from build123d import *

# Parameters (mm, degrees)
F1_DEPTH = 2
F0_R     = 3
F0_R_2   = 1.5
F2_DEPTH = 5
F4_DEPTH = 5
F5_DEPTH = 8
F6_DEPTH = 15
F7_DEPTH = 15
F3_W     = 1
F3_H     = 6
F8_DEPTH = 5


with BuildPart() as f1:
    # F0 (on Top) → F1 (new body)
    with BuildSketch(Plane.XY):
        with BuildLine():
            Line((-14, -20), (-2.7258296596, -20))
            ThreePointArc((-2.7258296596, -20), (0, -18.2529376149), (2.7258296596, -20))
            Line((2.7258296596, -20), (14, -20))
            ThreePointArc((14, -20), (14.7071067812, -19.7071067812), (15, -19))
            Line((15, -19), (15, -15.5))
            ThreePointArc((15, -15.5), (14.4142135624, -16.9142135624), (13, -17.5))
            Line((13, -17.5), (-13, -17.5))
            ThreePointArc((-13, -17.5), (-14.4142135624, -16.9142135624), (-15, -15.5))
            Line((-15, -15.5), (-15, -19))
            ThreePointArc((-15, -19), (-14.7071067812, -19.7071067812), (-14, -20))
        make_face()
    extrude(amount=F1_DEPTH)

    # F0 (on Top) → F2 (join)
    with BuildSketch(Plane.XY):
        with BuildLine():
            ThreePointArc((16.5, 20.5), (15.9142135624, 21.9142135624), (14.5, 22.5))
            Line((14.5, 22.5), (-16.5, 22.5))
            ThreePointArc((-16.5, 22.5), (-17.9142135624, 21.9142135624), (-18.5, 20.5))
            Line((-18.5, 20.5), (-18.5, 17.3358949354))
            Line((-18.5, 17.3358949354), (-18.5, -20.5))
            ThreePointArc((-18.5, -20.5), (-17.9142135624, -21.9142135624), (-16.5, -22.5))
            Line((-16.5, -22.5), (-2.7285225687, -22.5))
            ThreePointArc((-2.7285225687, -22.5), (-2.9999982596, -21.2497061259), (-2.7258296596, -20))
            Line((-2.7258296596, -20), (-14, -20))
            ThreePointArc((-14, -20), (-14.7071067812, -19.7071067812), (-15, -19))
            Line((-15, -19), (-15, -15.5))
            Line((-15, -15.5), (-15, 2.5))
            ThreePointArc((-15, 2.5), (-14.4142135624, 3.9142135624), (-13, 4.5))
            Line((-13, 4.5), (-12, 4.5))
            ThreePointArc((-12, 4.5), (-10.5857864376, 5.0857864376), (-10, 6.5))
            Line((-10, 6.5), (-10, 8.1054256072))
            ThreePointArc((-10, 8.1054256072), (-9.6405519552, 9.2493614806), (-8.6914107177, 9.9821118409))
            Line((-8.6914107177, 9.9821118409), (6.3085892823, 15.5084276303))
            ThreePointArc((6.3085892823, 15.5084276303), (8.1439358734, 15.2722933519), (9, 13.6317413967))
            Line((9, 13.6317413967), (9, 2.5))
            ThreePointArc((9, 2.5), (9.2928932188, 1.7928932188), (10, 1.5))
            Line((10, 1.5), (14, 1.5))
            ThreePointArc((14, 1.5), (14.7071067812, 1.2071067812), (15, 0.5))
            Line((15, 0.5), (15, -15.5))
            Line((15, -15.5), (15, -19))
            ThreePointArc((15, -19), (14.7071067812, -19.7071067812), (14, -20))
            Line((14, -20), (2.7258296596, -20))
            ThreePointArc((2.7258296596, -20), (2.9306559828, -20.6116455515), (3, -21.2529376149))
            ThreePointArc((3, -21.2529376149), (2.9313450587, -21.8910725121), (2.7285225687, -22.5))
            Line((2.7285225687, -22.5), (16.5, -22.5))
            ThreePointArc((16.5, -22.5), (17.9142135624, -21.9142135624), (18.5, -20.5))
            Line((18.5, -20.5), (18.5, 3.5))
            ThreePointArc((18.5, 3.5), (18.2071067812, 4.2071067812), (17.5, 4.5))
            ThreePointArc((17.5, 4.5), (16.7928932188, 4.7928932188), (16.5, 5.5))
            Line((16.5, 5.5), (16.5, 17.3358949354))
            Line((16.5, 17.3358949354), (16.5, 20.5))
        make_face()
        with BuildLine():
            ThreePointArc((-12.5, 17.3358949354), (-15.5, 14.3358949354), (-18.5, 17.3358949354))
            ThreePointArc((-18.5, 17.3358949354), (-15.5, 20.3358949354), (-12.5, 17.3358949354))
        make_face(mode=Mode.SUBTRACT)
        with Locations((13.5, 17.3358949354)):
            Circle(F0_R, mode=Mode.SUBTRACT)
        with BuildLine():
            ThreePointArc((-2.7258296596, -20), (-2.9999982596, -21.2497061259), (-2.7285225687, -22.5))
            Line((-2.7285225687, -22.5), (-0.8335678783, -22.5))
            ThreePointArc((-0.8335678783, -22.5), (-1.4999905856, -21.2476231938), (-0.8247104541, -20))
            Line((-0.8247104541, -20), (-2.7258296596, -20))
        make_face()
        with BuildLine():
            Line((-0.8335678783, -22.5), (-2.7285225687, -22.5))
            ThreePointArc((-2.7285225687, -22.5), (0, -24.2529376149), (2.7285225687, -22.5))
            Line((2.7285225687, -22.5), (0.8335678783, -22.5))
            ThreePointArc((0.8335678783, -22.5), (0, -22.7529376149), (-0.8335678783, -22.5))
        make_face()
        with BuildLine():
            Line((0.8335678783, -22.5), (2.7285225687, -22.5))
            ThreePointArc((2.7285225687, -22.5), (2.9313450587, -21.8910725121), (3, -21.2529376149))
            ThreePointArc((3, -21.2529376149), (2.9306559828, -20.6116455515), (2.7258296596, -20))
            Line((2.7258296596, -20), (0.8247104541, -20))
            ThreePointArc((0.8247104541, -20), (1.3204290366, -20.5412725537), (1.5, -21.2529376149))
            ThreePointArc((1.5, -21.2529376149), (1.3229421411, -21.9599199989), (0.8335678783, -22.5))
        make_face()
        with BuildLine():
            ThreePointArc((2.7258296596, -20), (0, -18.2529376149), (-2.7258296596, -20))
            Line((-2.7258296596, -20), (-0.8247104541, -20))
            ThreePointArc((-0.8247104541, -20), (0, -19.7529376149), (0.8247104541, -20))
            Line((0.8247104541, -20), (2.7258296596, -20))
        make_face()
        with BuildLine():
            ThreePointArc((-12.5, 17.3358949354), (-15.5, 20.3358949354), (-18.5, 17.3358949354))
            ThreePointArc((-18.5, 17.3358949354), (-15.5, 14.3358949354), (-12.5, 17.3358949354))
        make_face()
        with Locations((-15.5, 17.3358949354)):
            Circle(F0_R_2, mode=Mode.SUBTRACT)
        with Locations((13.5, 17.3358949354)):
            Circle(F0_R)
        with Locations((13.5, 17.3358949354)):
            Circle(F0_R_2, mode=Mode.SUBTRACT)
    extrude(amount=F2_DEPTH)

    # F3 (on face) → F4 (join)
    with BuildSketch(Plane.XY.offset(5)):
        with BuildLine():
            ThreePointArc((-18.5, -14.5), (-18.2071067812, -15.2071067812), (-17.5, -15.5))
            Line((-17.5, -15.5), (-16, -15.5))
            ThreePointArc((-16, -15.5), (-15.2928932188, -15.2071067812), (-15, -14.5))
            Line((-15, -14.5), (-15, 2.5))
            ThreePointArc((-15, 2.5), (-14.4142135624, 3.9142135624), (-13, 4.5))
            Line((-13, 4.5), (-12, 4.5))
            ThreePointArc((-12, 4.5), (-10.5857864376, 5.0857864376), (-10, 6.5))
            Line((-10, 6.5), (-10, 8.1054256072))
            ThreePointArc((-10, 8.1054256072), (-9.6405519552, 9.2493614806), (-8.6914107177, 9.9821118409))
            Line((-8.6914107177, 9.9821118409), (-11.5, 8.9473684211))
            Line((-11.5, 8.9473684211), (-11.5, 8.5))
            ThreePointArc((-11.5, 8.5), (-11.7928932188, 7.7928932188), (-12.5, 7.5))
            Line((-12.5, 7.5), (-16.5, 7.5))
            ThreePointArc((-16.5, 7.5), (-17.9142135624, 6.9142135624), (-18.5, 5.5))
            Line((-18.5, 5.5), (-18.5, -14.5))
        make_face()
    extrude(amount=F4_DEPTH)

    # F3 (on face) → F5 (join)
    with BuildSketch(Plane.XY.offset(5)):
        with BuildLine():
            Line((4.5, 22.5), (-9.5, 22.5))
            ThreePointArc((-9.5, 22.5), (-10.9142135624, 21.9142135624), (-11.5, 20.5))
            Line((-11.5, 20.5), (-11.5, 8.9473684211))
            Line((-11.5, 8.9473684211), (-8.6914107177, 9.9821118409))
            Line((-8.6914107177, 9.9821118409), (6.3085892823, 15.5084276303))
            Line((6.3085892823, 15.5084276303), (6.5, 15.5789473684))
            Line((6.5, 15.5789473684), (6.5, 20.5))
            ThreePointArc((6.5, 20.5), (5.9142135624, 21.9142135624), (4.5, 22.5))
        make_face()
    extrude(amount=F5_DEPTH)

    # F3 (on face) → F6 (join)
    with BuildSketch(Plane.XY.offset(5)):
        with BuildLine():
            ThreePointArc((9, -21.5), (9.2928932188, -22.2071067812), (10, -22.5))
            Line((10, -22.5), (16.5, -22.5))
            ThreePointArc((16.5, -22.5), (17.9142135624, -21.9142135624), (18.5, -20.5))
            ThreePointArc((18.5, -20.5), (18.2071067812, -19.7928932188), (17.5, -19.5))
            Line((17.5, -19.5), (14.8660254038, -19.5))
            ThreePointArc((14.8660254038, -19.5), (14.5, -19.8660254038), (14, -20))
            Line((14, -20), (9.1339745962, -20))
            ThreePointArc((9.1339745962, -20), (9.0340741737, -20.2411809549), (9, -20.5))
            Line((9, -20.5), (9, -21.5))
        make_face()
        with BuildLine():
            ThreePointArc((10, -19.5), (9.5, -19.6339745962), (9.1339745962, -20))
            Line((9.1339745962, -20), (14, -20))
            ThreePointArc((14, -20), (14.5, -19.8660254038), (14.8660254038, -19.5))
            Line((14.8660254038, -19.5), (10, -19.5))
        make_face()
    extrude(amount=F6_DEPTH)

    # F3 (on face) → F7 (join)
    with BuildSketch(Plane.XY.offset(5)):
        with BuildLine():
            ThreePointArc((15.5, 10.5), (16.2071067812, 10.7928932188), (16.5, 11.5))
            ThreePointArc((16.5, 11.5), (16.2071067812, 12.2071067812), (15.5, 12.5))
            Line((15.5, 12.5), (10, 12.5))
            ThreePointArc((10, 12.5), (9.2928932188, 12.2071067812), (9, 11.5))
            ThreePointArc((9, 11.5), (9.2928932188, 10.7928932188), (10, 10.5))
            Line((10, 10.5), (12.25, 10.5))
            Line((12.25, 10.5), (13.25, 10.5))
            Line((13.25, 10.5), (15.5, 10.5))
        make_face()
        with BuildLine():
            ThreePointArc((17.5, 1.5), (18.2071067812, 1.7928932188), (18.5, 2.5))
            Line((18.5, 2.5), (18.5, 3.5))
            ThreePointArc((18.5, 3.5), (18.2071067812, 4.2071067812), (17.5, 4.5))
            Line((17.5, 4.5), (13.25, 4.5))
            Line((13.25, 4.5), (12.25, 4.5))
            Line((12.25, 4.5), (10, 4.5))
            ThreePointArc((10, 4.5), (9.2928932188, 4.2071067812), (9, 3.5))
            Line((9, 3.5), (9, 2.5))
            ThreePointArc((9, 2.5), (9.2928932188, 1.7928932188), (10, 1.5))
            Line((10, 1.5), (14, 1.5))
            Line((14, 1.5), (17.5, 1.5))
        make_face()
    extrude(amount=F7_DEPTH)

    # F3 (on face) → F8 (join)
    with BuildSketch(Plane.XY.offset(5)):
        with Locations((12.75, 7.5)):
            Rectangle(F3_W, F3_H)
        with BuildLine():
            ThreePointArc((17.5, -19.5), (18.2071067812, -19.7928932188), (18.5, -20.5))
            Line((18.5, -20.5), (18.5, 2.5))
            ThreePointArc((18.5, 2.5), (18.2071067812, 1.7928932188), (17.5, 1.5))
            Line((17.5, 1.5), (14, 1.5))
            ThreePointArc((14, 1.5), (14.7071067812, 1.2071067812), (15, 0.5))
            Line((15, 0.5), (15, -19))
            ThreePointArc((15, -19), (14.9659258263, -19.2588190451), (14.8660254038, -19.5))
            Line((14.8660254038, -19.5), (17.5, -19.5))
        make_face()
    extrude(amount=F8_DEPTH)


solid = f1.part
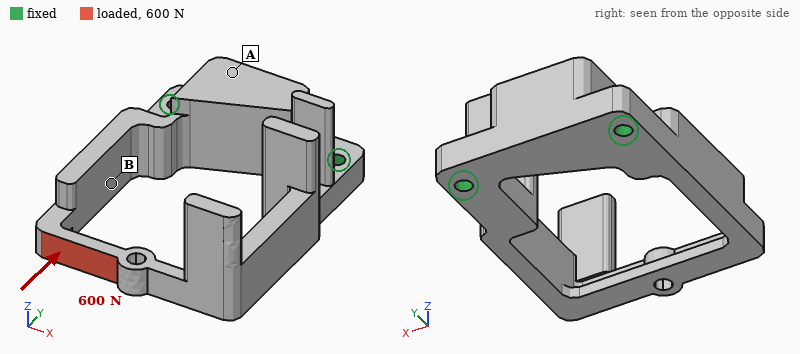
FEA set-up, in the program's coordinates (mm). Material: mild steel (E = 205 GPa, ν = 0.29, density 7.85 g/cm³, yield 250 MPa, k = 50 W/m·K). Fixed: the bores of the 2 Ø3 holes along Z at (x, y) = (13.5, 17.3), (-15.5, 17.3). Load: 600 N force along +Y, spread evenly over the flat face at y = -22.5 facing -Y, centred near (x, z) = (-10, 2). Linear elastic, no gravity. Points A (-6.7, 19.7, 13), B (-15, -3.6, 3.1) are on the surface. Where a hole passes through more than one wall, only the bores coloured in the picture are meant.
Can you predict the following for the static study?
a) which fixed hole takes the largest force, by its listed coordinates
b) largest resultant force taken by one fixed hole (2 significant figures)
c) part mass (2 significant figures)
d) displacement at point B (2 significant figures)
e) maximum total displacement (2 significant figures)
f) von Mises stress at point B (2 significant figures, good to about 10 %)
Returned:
(-15.5, 17.3)
500 N
57 g
5.1 µm
28 µm
37 MPa
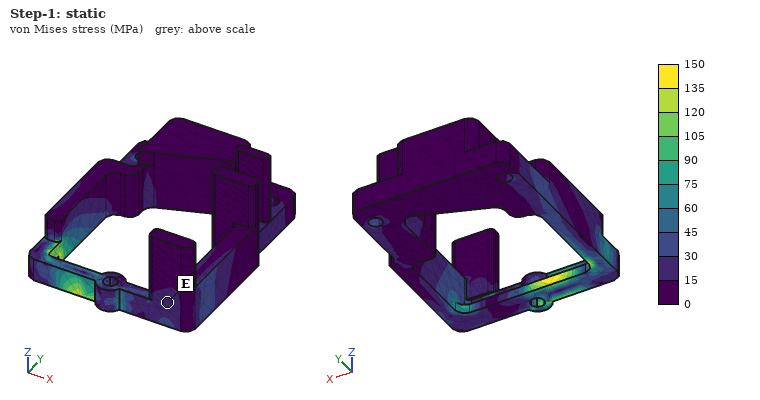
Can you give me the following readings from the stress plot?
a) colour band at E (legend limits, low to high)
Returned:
15 to 30 MPa
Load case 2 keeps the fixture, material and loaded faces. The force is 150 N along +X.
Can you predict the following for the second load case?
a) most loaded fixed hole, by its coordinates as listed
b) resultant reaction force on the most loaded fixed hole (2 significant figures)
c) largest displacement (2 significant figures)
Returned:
(13.5, 17.3)
200 N
36 µm
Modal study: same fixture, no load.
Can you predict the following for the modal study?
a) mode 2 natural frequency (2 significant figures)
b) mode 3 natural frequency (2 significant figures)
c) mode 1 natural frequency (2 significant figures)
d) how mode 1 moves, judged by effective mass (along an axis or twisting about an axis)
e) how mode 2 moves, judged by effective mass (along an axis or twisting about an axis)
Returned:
3000 Hz
4100 Hz
2100 Hz
along Z
along X
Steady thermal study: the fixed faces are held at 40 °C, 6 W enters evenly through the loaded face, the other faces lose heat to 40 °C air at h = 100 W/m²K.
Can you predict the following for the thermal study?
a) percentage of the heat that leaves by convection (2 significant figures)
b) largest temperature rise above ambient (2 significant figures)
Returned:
74 %
54 K
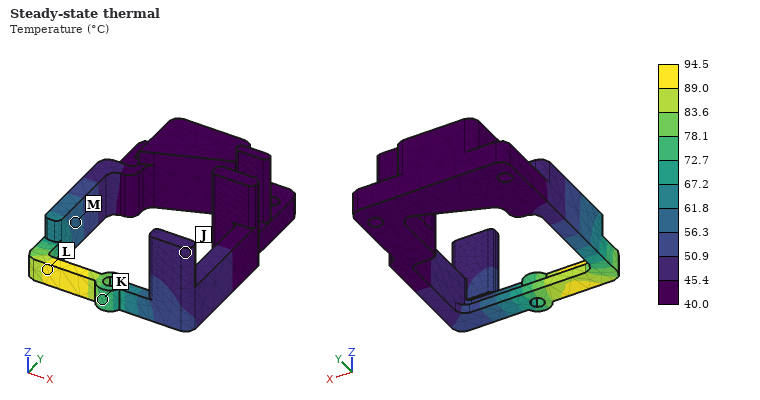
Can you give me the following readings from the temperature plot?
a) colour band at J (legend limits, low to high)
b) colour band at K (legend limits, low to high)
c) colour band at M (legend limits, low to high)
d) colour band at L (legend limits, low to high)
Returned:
45.4 to 50.9 °C
72.7 to 78.1 °C
56.3 to 61.8 °C
89.0 to 94.5 °C
